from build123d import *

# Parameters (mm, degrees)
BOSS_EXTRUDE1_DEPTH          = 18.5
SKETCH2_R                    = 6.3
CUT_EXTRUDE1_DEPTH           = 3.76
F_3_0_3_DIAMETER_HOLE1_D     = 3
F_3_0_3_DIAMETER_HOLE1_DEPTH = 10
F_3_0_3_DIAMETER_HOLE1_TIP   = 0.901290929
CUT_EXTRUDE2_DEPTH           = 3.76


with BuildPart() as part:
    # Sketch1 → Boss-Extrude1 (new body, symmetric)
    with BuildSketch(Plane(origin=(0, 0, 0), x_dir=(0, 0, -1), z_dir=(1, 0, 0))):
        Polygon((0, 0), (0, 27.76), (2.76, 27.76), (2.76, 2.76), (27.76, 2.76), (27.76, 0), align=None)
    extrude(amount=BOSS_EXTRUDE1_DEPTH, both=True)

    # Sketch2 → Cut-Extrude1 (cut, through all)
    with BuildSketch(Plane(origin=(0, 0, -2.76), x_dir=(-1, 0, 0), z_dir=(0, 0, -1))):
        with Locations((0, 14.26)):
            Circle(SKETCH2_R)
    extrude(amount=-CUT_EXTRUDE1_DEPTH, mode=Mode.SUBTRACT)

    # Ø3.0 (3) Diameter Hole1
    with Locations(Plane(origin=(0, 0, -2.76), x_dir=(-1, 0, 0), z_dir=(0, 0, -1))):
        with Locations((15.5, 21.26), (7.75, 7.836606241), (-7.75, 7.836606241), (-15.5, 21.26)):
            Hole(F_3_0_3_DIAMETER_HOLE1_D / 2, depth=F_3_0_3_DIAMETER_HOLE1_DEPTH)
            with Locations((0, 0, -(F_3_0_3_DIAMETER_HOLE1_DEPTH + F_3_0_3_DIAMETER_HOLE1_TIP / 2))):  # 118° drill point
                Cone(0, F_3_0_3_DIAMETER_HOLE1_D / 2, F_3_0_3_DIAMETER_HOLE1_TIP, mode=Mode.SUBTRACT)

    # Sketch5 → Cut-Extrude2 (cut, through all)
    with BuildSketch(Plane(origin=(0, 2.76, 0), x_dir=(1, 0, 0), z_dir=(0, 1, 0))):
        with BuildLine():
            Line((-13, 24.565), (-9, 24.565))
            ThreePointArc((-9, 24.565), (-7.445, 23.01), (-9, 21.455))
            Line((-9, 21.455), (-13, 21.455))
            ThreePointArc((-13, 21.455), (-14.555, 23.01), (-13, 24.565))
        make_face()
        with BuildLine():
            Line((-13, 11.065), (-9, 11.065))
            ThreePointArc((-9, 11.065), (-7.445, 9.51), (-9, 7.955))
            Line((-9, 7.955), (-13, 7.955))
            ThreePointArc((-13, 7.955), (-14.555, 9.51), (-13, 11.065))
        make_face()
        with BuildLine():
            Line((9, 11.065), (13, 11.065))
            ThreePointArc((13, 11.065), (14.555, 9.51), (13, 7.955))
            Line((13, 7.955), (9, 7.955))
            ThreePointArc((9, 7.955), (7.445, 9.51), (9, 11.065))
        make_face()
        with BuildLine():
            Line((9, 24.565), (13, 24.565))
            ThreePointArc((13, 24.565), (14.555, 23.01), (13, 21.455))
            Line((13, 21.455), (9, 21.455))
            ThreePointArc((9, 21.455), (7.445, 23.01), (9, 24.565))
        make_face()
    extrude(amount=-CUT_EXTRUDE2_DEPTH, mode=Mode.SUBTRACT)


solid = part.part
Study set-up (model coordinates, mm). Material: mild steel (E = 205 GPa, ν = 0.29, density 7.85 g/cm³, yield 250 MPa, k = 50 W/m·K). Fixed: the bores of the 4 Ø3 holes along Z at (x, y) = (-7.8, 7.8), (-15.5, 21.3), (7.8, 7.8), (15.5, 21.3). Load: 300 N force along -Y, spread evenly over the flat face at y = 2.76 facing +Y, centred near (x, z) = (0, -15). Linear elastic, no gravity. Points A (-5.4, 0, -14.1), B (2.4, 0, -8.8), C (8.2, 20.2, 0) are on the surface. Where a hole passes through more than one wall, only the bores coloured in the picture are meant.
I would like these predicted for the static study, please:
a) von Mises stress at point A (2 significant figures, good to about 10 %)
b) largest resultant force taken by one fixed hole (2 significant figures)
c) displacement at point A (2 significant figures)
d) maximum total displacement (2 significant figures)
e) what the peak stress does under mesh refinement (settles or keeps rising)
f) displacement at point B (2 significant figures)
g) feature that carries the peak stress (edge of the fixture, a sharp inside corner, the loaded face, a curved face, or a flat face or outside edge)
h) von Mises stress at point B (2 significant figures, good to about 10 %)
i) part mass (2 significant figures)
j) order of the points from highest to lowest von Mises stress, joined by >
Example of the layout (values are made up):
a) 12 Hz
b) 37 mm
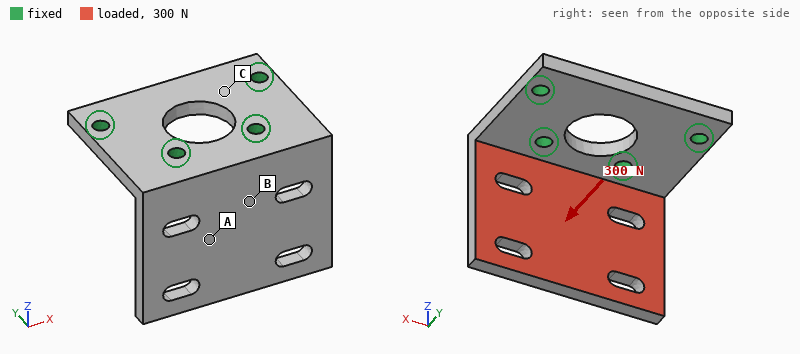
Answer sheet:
a) 25 MPa
b) 140 N
c) 0.046 mm
d) 0.11 mm
e) keeps rising
f) 0.025 mm
g) edge of the fixture
h) 56 MPa
i) 37 g
j) B > A > C
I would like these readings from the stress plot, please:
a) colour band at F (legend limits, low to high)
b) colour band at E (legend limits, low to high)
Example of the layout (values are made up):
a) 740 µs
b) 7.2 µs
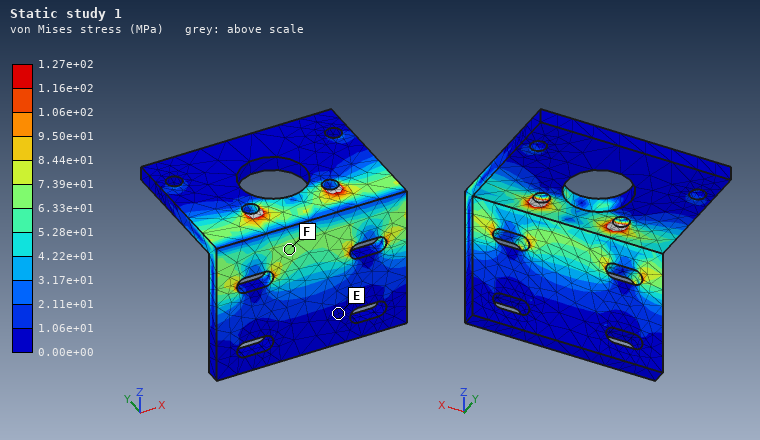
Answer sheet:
a) 6.33e+01 to 7.39e+01 MPa
b) 0.00e+00 to 1.06e+01 MPa
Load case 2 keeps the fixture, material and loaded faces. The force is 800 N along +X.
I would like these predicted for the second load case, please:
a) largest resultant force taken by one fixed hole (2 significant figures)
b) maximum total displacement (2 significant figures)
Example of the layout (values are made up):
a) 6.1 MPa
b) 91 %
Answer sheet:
a) 730 N
b) 43 µm
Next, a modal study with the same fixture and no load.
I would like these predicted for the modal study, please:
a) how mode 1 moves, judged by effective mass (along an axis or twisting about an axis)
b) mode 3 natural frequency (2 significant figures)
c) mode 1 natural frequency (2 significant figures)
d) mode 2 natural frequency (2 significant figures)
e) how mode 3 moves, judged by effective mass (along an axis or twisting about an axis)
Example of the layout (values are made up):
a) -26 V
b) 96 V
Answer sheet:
a) along Y
b) 7500 Hz
c) 2400 Hz
d) 5100 Hz
e) along X
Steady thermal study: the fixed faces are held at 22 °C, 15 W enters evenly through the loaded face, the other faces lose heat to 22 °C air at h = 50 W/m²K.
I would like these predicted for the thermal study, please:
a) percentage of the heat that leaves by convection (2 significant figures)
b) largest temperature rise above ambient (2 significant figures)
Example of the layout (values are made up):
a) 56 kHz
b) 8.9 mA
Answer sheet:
a) 22 %
b) 56 K
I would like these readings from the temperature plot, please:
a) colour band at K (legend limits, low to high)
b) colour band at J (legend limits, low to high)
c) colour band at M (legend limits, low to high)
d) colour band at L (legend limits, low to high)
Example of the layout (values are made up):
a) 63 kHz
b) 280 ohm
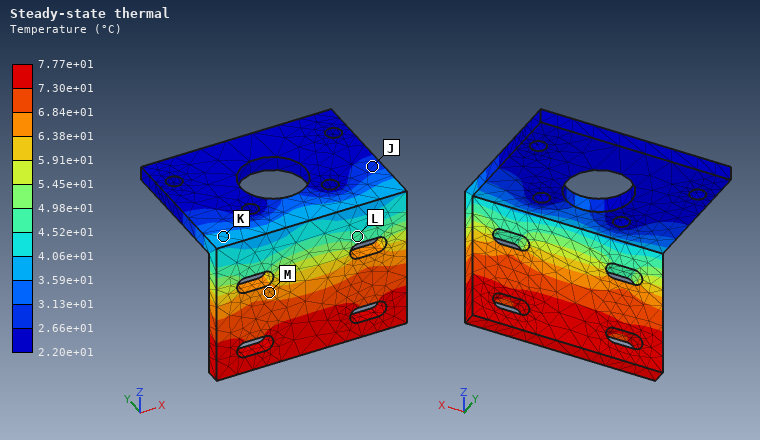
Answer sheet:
a) 3.59e+01 to 4.06e+01 °C
b) 2.66e+01 to 3.13e+01 °C
c) 6.38e+01 to 6.84e+01 °C
d) 4.52e+01 to 4.98e+01 °C
